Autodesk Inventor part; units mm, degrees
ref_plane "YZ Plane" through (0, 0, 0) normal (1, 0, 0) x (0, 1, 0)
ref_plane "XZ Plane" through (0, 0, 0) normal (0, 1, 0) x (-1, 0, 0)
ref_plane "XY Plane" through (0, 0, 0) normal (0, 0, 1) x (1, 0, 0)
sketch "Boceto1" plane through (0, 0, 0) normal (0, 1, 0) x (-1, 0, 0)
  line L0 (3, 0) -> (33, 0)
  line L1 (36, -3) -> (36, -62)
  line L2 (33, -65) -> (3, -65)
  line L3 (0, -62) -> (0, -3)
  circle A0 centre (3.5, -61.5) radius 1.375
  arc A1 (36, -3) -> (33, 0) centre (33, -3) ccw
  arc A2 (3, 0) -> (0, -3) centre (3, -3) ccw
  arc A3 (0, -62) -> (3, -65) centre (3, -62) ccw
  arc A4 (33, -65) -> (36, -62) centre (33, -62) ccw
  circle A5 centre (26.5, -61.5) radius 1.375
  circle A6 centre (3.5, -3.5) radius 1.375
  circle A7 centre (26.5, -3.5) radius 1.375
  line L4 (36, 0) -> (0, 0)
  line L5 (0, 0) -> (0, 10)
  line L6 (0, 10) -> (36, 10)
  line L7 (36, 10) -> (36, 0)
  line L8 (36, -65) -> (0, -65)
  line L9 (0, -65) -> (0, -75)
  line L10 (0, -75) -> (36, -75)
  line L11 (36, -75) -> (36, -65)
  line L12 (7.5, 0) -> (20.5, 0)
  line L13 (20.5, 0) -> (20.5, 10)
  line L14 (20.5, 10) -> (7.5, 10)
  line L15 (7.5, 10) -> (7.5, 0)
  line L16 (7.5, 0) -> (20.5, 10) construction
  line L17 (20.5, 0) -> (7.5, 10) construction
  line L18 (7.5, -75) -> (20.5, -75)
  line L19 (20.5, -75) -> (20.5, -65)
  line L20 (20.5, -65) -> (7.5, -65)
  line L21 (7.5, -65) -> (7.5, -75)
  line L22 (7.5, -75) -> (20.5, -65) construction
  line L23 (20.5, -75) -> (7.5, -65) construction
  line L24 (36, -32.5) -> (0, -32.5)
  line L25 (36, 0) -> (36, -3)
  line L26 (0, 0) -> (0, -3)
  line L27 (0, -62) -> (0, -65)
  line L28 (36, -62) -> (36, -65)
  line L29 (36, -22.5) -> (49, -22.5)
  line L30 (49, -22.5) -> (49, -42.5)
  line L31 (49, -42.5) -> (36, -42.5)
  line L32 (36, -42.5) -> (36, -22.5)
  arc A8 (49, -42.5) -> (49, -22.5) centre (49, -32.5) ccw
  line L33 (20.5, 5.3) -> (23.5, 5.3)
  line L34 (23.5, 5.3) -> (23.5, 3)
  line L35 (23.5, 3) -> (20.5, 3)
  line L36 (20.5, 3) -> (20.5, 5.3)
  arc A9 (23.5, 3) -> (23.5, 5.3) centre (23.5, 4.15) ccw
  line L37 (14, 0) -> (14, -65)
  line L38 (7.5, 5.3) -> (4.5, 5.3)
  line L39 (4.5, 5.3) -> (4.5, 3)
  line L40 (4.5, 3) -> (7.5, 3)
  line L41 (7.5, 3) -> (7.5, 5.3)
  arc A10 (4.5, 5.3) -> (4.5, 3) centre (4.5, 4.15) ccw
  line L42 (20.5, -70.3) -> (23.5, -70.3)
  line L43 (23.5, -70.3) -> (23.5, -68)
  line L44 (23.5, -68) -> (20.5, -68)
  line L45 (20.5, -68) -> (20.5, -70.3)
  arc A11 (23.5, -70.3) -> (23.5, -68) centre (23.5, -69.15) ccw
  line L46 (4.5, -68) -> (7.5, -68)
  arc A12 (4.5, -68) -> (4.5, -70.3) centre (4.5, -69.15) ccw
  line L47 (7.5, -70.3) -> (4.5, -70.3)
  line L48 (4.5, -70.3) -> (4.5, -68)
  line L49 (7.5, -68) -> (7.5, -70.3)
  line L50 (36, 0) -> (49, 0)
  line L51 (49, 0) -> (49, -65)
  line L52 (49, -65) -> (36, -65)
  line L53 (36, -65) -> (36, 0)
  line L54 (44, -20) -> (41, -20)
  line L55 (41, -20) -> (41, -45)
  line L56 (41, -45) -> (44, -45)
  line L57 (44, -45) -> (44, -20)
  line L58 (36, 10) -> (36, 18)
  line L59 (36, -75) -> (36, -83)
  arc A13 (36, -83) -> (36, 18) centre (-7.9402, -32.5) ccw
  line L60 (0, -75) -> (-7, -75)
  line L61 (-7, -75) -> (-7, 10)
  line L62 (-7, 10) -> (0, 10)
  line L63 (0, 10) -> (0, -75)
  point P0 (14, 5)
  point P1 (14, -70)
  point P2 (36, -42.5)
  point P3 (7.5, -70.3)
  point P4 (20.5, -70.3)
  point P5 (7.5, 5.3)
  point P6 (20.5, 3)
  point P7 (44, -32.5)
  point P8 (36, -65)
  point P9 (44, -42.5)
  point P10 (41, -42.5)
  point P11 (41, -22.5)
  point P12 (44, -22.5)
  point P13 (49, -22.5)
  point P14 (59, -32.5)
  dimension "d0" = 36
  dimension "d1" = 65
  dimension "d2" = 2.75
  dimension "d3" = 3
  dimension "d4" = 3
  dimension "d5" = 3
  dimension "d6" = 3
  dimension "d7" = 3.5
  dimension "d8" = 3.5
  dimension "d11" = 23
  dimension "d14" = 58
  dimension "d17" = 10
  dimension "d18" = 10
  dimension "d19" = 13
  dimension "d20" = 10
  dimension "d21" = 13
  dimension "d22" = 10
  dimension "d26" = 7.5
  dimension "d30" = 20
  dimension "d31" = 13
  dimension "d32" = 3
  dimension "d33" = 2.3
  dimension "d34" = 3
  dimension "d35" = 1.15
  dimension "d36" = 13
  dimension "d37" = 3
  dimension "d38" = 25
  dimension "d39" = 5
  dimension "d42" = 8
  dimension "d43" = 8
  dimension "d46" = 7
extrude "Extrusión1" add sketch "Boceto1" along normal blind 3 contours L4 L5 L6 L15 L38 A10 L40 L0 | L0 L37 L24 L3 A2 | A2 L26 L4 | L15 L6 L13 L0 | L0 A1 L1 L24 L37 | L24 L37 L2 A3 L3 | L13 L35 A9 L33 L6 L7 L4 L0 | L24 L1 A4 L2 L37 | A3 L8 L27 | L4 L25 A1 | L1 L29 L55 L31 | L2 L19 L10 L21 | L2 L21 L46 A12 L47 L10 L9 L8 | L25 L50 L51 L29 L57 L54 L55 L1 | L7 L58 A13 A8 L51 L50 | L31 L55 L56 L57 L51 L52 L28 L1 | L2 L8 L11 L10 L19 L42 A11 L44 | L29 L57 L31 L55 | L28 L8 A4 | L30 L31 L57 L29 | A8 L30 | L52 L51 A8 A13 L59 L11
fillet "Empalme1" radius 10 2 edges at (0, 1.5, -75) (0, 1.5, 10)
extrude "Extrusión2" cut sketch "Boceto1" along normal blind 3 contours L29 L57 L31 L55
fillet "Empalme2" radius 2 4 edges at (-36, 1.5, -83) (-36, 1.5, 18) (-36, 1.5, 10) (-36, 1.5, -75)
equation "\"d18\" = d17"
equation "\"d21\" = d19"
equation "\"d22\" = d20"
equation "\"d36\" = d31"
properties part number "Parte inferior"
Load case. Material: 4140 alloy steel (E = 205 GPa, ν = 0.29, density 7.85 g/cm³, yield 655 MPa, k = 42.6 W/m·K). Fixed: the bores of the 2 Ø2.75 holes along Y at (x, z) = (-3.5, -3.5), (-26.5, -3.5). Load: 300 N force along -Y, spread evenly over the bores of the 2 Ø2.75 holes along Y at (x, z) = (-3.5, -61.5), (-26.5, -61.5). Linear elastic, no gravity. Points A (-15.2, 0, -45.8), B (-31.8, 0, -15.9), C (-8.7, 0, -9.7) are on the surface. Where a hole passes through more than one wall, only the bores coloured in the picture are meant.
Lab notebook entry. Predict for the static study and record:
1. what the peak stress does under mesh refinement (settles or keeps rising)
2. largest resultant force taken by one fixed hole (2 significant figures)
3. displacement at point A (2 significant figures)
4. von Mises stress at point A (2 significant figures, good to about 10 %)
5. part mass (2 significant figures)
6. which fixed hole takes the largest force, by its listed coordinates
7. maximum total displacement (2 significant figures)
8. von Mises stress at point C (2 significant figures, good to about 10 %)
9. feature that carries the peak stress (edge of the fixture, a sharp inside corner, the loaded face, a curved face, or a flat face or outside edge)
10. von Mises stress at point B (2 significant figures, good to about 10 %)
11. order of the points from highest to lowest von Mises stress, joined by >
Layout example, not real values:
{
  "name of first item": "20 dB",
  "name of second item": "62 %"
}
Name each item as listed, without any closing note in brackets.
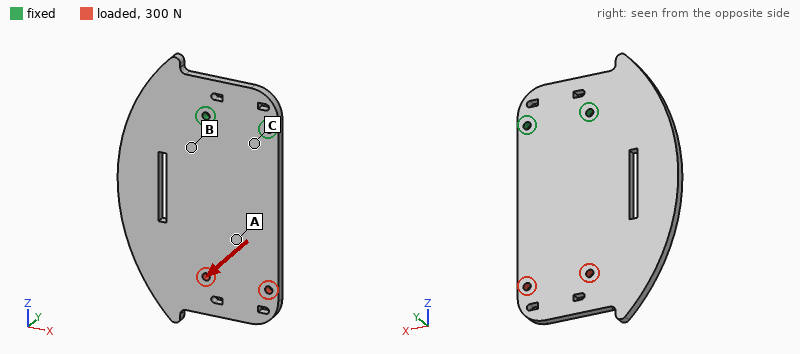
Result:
{
  "what the peak stress does under mesh refinement": "keeps rising",
  "largest resultant force taken by one fixed hole": "160 N",
  "displacement at point A": "0.59 mm",
  "von Mises stress at point A": "65 MPa",
  "part mass": "110 g",
  "which fixed hole takes the largest force, by its listed coordinates": "(-26.5, -3.5)",
  "maximum total displacement": "1.3 mm",
  "von Mises stress at point C": "210 MPa",
  "feature that carries the peak stress": "edge of the fixture",
  "von Mises stress at point B": "150 MPa",
  "order of the points from highest to lowest von Mises stress, joined by >": "C > B > A"
}
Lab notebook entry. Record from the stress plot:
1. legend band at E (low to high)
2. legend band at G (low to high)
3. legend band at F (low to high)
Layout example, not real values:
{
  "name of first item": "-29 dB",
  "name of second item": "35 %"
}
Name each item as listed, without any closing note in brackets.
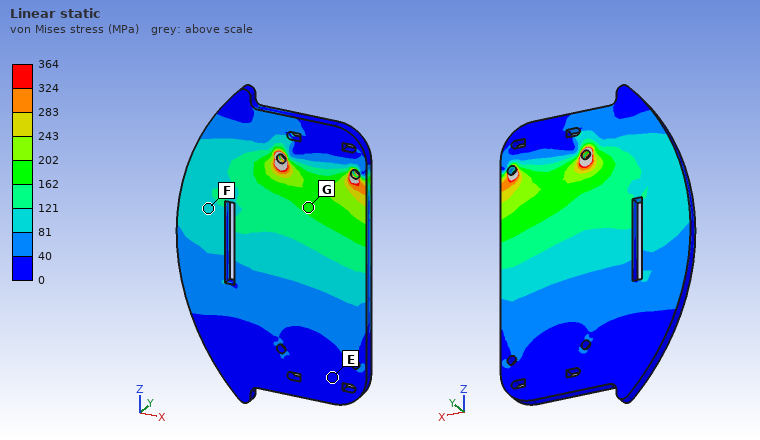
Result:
{
  "legend band at E": "0 to 40 MPa",
  "legend band at G": "162 to 202 MPa",
  "legend band at F": "81 to 121 MPa"
}
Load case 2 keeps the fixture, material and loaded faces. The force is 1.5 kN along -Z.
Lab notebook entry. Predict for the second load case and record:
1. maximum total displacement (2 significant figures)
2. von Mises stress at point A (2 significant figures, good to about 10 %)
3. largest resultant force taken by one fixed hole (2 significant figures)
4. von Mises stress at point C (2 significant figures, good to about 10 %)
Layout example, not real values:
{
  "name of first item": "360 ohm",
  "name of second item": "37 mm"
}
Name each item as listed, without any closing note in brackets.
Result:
{
  "maximum total displacement": "7.7 µm",
  "von Mises stress at point A": "13 MPa",
  "largest resultant force taken by one fixed hole": "760 N",
  "von Mises stress at point C": "15 MPa"
}
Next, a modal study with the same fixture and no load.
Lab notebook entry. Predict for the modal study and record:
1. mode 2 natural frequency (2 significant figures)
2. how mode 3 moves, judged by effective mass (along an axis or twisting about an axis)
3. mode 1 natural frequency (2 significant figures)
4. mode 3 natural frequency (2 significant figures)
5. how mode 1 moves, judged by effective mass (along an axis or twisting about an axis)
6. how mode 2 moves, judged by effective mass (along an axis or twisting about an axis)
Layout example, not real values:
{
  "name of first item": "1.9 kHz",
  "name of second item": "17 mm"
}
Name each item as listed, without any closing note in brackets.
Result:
{
  "mode 2 natural frequency": "1300 Hz",
  "how mode 3 moves, judged by effective mass": "along Y",
  "mode 1 natural frequency": "450 Hz",
  "mode 3 natural frequency": "2600 Hz",
  "how mode 1 moves, judged by effective mass": "along Y",
  "how mode 2 moves, judged by effective mass": "twisting about Z"
}
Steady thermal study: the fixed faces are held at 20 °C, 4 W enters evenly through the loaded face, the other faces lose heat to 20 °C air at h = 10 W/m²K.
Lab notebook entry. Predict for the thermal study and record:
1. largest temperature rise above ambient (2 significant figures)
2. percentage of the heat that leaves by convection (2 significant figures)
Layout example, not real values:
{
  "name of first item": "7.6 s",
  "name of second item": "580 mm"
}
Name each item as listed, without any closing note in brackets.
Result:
{
  "largest temperature rise above ambient": "37 K",
  "percentage of the heat that leaves by convection": "37 %"
}
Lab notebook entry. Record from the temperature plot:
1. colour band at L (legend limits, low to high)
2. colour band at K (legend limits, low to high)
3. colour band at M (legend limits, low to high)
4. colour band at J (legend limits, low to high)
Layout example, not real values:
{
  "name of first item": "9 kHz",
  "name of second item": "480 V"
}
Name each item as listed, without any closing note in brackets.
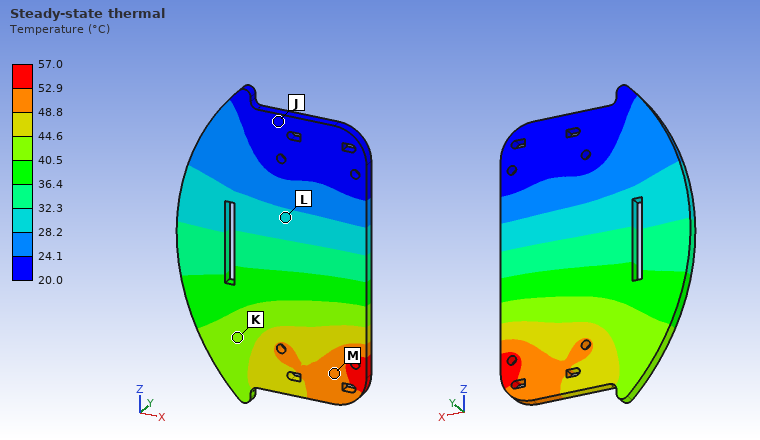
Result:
{
  "colour band at L": "28.2 to 32.3 °C",
  "colour band at K": "40.5 to 44.6 °C",
  "colour band at M": "48.8 to 52.9 °C",
  "colour band at J": "20.0 to 24.1 °C"
}
